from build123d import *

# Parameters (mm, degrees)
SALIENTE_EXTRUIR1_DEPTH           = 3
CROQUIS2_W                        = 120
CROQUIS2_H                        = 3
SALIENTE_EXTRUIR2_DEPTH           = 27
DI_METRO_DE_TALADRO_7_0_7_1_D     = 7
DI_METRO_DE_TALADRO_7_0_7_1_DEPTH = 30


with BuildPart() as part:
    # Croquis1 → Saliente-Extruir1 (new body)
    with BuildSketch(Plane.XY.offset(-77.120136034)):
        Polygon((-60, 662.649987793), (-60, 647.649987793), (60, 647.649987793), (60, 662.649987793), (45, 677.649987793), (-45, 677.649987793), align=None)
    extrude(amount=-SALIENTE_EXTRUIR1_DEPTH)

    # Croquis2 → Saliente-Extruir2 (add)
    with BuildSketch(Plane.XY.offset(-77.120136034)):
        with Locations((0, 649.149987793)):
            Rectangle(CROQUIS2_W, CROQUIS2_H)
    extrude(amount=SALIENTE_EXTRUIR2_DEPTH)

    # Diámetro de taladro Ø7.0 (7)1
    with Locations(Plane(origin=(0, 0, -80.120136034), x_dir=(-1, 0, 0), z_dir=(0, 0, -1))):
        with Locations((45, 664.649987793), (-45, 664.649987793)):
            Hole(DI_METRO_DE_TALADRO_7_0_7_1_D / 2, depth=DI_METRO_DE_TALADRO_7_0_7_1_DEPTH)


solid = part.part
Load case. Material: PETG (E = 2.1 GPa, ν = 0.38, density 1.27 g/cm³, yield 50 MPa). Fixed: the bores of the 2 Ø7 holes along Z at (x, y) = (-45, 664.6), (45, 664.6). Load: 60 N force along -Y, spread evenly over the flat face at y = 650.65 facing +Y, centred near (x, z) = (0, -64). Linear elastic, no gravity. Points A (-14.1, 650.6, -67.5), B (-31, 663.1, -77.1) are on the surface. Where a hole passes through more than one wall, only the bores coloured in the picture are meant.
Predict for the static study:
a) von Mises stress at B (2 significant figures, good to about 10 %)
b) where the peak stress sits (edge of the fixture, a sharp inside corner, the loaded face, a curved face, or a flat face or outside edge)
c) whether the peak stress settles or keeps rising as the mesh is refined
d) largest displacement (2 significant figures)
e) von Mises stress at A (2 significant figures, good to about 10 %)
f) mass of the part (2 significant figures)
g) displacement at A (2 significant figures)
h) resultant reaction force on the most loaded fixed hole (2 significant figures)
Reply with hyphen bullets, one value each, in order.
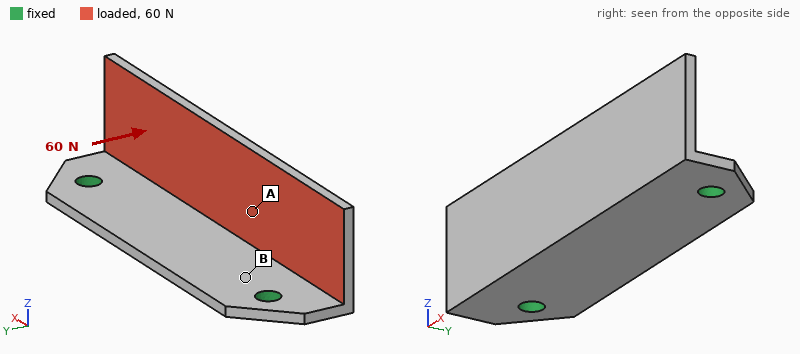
- 4.0 MPa
- edge of the fixture
- keeps rising
- 1.2 mm
- 1.5 MPa
- 25 g
- 0.46 mm
- 30 N
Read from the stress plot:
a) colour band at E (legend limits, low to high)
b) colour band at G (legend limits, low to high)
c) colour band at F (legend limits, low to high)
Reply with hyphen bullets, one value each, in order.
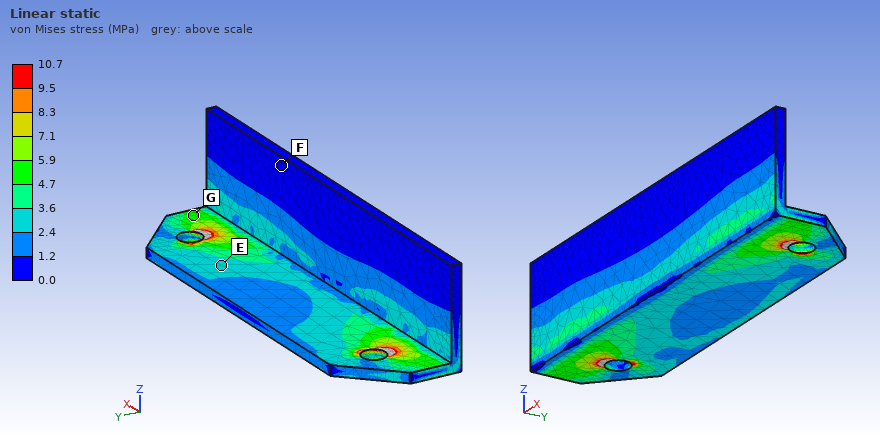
- 2.4 to 3.6 MPa
- 4.7 to 5.9 MPa
- 0.0 to 1.2 MPa
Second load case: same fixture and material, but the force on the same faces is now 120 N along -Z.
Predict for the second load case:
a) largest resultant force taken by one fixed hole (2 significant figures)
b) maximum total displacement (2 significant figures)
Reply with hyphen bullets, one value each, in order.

- 62 N
- 0.80 mm
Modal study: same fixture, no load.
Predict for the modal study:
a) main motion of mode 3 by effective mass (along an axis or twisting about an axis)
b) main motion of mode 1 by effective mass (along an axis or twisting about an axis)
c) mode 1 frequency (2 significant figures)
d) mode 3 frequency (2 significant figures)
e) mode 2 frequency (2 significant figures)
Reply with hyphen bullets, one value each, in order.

- along Z
- along Y
- 370 Hz
- 740 Hz
- 550 Hz
